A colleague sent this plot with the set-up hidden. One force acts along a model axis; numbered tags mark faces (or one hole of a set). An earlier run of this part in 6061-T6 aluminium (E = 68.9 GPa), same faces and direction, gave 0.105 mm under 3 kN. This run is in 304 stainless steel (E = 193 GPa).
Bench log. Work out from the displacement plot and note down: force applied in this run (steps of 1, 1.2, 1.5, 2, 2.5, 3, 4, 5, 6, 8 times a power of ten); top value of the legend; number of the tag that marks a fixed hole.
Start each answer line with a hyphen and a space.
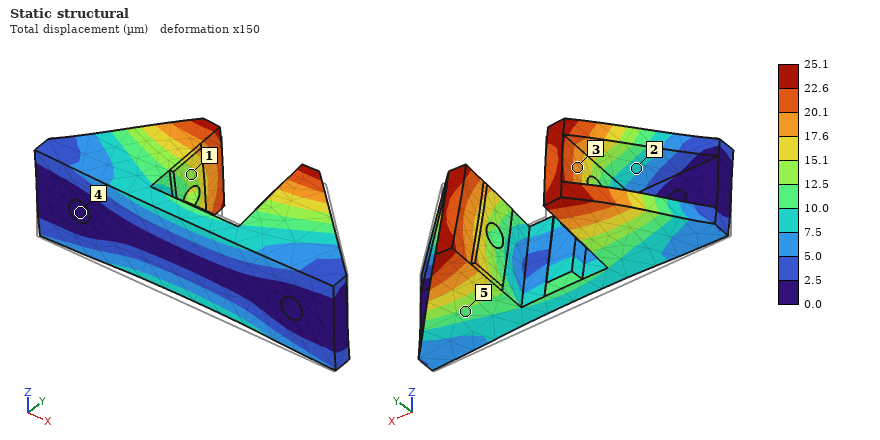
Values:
- 2 kN
- 25.1 µm
- 4
